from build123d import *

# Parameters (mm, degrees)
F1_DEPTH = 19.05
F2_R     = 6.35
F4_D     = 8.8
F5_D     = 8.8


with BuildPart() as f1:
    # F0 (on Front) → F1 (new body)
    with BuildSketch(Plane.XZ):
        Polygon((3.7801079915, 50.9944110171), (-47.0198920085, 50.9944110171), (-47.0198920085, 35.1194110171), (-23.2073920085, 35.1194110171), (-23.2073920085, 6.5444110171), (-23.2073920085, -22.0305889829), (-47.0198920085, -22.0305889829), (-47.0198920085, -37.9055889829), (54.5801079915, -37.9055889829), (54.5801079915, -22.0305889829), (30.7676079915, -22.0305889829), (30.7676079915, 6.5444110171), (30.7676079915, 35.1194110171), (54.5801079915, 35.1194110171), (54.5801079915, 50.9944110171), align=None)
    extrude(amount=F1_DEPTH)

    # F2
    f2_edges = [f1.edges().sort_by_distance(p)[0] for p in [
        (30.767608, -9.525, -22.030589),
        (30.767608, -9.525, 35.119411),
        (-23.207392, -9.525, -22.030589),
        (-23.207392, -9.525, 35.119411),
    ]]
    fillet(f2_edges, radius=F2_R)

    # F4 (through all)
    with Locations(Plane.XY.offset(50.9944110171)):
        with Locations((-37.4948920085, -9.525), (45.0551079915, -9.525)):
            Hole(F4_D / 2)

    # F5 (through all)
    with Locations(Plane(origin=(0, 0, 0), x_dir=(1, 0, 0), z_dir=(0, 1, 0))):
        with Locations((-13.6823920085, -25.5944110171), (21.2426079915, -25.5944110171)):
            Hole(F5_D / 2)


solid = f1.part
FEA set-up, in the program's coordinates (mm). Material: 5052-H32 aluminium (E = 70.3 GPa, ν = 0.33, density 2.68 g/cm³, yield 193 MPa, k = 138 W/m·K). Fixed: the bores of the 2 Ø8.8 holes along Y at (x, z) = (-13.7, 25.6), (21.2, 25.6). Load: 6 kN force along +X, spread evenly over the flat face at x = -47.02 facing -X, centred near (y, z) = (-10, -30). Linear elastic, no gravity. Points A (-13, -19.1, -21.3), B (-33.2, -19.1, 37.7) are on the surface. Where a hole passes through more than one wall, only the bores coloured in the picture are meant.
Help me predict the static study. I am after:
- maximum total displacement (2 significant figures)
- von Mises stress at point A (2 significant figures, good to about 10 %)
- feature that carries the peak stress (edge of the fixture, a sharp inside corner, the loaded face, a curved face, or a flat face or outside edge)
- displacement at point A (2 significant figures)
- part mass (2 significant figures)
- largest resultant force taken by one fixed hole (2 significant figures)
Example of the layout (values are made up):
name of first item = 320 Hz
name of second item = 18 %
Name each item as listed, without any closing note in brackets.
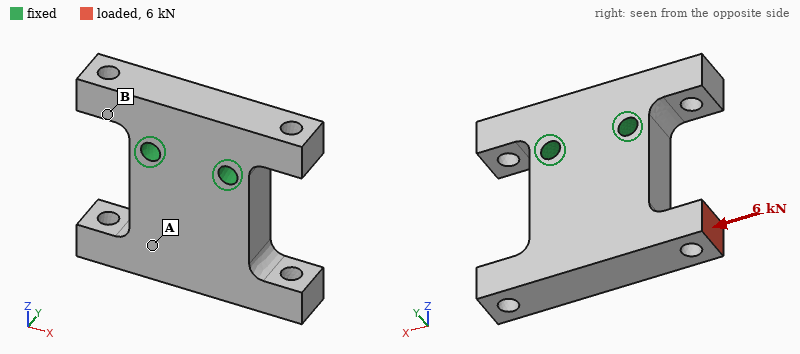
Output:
maximum total displacement = 70 µm
von Mises stress at point A = 16 MPa
feature that carries the peak stress = a curved face
displacement at point A = 28 µm
part mass = 310 g
largest resultant force taken by one fixed hole = 8.9 kN
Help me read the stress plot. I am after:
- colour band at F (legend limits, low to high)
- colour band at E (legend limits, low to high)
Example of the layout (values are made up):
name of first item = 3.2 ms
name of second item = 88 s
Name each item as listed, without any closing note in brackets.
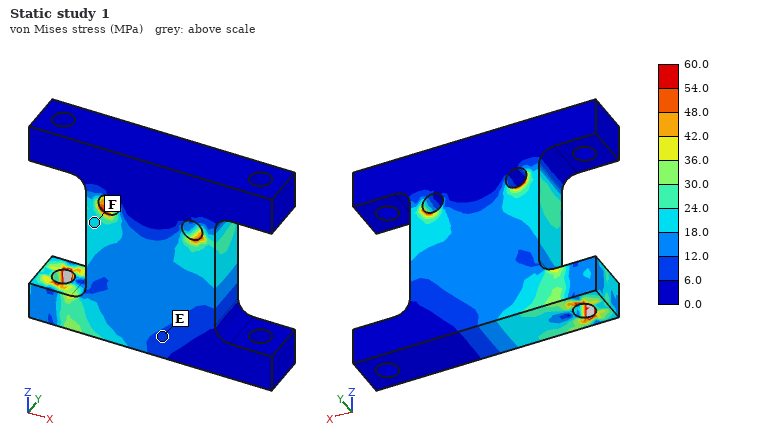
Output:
colour band at F = 18.0 to 24.0 MPa
colour band at E = 6.0 to 12.0 MPa
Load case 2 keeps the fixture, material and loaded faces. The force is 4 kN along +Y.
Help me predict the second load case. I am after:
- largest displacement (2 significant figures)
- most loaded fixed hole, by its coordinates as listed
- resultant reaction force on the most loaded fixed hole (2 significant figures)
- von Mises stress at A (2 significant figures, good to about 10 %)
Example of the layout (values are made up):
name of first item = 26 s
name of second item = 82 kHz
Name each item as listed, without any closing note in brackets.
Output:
largest displacement = 0.43 mm
most loaded fixed hole, by its coordinates as listed = (-13.7, 25.6)
resultant reaction force on the most loaded fixed hole = 6.5 kN
von Mises stress at A = 95 MPa
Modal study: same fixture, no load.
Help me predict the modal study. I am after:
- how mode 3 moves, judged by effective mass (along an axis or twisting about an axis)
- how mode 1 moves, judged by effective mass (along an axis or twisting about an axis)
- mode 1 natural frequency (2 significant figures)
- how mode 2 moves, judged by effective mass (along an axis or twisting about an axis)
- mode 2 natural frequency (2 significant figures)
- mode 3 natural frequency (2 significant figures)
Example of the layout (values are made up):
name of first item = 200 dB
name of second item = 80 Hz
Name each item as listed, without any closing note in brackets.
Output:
how mode 3 moves, judged by effective mass = along X
how mode 1 moves, judged by effective mass = along Y
mode 1 natural frequency = 3000 Hz
how mode 2 moves, judged by effective mass = twisting about Z
mode 2 natural frequency = 4500 Hz
mode 3 natural frequency = 6000 Hz
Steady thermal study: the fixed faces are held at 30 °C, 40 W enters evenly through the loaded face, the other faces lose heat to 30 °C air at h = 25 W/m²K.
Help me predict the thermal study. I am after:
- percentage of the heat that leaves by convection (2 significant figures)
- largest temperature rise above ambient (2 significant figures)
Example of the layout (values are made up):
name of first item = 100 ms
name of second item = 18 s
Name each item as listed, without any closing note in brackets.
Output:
percentage of the heat that leaves by convection = 11 %
largest temperature rise above ambient = 52 K
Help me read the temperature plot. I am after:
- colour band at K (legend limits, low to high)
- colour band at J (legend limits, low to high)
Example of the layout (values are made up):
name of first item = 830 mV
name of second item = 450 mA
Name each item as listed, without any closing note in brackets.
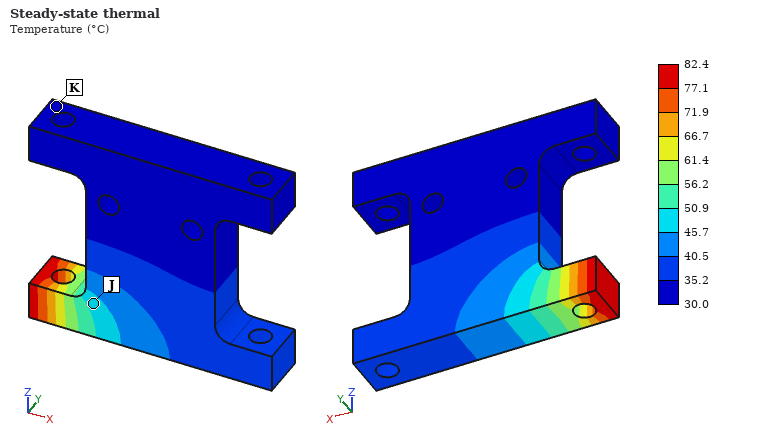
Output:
colour band at K = 30.0 to 35.2 °C
colour band at J = 45.7 to 50.9 °C
